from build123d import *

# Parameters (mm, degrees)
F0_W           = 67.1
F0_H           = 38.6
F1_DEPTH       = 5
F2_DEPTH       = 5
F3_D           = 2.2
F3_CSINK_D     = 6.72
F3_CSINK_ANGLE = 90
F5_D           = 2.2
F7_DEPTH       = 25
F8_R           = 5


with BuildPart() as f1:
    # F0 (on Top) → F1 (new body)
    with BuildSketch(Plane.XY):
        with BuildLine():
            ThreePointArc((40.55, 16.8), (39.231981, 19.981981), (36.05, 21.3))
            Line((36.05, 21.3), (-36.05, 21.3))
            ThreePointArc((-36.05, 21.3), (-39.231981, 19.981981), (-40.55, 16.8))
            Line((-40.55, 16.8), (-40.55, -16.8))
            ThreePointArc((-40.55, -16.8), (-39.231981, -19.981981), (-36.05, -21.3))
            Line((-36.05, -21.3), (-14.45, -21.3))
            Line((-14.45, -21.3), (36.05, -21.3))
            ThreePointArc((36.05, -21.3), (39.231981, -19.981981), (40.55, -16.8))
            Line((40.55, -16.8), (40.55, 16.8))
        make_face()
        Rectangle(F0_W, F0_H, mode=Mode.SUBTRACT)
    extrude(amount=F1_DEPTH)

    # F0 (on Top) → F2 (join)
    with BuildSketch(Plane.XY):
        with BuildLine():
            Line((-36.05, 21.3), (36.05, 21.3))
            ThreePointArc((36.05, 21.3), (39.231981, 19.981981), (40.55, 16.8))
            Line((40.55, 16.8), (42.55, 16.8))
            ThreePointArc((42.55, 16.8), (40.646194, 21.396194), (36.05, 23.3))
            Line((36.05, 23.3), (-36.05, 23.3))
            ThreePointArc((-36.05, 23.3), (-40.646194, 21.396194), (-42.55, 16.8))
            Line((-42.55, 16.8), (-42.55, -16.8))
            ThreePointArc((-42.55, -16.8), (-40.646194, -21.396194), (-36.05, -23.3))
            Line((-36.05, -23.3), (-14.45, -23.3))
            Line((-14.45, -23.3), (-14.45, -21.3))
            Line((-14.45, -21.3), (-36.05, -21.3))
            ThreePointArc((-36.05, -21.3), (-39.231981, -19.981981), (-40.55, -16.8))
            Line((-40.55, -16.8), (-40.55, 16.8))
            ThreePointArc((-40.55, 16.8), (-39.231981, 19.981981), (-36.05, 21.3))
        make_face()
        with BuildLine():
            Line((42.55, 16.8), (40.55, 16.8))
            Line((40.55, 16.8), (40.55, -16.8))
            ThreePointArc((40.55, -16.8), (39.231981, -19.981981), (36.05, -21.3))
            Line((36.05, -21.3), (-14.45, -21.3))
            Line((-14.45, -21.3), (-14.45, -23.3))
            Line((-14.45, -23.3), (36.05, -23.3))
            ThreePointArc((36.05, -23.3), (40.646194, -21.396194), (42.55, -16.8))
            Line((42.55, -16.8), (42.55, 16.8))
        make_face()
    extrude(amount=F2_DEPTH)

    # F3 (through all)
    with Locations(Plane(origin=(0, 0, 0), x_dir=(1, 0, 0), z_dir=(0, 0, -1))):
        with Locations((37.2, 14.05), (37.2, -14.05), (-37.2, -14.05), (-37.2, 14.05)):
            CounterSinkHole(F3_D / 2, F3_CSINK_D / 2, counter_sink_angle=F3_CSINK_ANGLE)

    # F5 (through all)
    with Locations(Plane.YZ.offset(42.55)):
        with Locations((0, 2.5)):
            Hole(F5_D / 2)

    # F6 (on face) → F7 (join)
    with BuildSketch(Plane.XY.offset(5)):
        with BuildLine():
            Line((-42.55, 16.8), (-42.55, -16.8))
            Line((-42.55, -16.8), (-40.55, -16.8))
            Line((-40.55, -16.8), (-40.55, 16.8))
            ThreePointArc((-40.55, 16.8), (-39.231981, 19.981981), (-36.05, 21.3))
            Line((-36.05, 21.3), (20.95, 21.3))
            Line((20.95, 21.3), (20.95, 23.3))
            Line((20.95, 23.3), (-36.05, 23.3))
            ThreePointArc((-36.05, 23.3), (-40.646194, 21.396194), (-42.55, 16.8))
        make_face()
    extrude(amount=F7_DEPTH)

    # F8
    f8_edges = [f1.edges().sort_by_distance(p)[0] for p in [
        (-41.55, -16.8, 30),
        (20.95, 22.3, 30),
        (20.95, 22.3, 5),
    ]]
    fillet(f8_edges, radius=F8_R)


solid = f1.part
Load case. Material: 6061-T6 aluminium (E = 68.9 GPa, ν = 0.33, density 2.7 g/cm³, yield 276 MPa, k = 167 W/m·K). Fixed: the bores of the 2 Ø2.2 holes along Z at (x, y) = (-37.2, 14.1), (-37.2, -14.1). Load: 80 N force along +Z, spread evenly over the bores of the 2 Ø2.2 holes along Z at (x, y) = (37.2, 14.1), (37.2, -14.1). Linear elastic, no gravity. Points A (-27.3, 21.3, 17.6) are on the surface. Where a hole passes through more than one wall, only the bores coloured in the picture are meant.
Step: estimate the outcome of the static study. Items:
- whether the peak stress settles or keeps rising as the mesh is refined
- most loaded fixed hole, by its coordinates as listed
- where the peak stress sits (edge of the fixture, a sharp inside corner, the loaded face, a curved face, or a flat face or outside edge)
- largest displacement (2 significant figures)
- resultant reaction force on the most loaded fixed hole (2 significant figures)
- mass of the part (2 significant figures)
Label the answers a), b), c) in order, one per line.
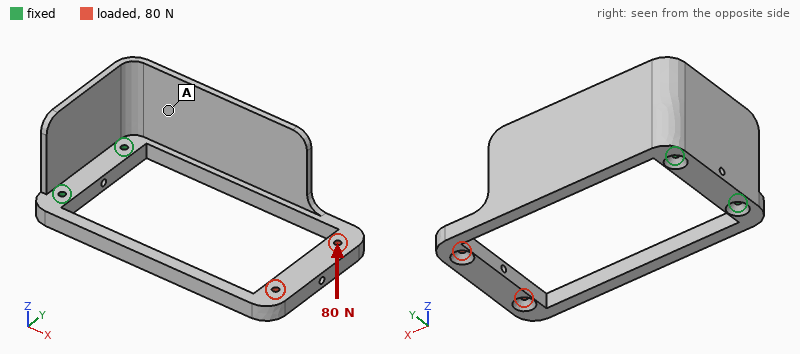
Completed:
a) keeps rising
b) (-37.2, -14.1)
c) edge of the fixture
d) 1.1 mm
e) 79 N
f) 31 g
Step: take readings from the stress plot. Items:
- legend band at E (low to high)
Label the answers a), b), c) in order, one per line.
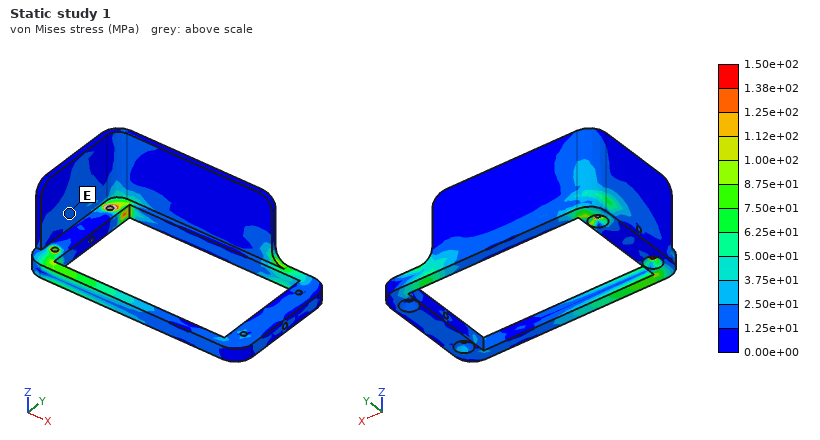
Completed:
a) 1.25e+01 to 2.50e+01 MPa
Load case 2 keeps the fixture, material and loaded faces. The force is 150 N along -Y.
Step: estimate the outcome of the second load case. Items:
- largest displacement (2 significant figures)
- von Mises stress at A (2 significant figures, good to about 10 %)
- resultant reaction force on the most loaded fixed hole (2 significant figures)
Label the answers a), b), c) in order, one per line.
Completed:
a) 1.2 mm
b) 44 MPa
c) 360 N
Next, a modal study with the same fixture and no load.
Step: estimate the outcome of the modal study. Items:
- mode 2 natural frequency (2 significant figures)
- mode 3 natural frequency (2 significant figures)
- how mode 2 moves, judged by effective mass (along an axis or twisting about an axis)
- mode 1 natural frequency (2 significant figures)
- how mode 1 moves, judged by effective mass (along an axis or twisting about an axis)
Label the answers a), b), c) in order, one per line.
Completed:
a) 580 Hz
b) 1100 Hz
c) along Y
d) 530 Hz
e) along Z
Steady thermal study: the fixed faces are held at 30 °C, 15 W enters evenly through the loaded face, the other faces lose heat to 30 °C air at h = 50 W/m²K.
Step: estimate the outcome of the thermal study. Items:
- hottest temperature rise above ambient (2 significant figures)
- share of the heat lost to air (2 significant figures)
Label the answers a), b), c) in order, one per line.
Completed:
a) 72 K
b) 64 %
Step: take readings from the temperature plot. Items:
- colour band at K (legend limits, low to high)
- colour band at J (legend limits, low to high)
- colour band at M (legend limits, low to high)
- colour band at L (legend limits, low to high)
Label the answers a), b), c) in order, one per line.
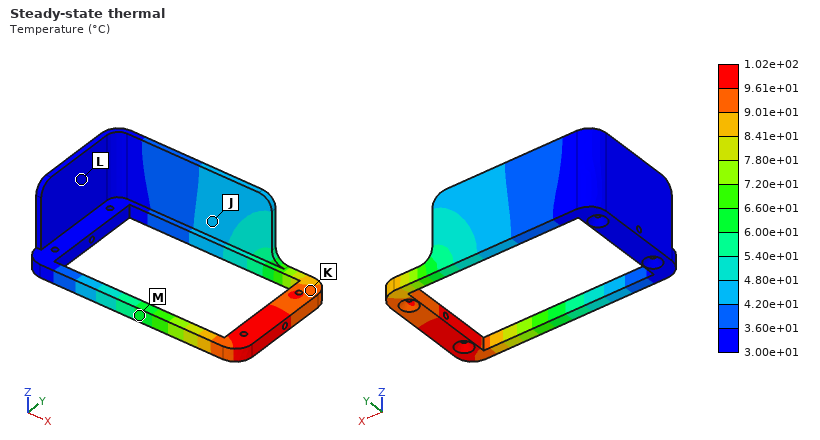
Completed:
a) 9.01e+01 to 9.61e+01 °C
b) 4.20e+01 to 4.80e+01 °C
c) 6.00e+01 to 6.60e+01 °C
d) 3.00e+01 to 3.60e+01 °C
